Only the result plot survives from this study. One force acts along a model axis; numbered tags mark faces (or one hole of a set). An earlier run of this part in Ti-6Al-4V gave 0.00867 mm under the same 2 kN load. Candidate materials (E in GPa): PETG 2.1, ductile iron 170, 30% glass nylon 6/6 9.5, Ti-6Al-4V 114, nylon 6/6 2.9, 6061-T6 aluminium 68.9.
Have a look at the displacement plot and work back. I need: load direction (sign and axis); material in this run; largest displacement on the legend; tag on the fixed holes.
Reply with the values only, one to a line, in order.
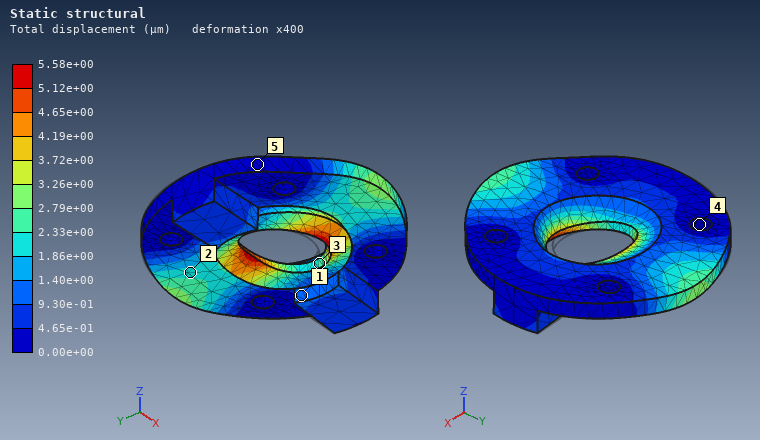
-Y
ductile iron
5.58e+00 µm
4
